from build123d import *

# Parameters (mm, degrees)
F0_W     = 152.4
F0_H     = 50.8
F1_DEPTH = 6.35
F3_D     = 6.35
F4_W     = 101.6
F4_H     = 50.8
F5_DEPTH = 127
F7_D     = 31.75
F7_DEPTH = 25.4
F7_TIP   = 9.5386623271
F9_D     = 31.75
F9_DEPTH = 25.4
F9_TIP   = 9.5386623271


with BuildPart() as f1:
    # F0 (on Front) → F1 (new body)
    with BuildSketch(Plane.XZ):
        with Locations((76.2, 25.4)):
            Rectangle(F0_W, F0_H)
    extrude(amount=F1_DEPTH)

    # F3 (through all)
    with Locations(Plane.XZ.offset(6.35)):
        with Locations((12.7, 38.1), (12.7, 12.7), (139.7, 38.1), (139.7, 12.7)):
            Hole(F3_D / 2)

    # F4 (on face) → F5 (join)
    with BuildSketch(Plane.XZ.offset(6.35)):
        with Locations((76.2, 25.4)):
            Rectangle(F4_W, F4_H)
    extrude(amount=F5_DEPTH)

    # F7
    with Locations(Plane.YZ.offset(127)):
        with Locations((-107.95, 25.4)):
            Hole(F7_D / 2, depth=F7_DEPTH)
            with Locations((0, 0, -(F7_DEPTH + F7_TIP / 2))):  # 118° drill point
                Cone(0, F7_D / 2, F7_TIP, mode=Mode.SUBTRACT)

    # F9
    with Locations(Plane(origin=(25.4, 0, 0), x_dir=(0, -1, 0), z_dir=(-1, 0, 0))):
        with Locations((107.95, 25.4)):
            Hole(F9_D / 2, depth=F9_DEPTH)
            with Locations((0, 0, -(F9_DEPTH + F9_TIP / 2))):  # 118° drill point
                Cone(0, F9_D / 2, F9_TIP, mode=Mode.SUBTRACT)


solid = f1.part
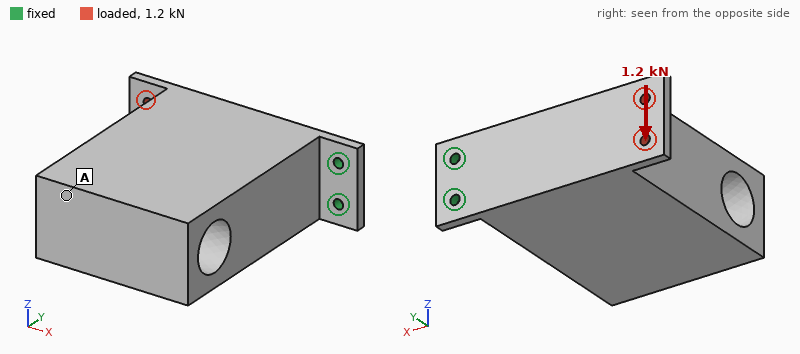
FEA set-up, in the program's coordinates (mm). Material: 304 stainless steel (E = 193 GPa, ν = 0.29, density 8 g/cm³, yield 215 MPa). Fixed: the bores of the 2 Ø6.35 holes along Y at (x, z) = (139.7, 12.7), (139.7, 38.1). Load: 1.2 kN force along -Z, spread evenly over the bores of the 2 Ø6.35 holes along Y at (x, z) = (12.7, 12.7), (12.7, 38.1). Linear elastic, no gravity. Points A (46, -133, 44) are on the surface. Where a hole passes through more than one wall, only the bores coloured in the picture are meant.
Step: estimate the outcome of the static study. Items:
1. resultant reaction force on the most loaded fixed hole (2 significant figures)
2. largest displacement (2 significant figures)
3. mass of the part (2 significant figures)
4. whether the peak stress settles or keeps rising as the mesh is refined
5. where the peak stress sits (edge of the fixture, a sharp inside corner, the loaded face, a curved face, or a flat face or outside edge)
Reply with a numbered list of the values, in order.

1. 5.2 kN
2. 57 µm
3. 5.3 kg
4. keeps rising
5. edge of the fixture
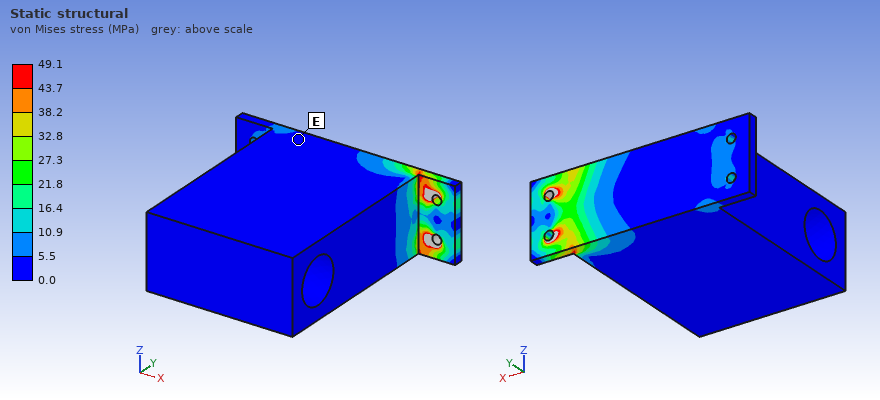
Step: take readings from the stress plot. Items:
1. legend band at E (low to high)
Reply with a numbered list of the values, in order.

1. 0.0 to 5.5 MPa
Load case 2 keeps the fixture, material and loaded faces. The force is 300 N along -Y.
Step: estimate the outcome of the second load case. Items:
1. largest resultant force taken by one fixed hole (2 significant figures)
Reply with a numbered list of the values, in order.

1. 150 N
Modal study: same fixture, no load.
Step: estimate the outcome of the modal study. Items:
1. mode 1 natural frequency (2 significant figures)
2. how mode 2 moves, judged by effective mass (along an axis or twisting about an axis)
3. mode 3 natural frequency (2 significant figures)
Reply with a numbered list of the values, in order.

1. 86 Hz
2. along Z
3. 910 Hz
